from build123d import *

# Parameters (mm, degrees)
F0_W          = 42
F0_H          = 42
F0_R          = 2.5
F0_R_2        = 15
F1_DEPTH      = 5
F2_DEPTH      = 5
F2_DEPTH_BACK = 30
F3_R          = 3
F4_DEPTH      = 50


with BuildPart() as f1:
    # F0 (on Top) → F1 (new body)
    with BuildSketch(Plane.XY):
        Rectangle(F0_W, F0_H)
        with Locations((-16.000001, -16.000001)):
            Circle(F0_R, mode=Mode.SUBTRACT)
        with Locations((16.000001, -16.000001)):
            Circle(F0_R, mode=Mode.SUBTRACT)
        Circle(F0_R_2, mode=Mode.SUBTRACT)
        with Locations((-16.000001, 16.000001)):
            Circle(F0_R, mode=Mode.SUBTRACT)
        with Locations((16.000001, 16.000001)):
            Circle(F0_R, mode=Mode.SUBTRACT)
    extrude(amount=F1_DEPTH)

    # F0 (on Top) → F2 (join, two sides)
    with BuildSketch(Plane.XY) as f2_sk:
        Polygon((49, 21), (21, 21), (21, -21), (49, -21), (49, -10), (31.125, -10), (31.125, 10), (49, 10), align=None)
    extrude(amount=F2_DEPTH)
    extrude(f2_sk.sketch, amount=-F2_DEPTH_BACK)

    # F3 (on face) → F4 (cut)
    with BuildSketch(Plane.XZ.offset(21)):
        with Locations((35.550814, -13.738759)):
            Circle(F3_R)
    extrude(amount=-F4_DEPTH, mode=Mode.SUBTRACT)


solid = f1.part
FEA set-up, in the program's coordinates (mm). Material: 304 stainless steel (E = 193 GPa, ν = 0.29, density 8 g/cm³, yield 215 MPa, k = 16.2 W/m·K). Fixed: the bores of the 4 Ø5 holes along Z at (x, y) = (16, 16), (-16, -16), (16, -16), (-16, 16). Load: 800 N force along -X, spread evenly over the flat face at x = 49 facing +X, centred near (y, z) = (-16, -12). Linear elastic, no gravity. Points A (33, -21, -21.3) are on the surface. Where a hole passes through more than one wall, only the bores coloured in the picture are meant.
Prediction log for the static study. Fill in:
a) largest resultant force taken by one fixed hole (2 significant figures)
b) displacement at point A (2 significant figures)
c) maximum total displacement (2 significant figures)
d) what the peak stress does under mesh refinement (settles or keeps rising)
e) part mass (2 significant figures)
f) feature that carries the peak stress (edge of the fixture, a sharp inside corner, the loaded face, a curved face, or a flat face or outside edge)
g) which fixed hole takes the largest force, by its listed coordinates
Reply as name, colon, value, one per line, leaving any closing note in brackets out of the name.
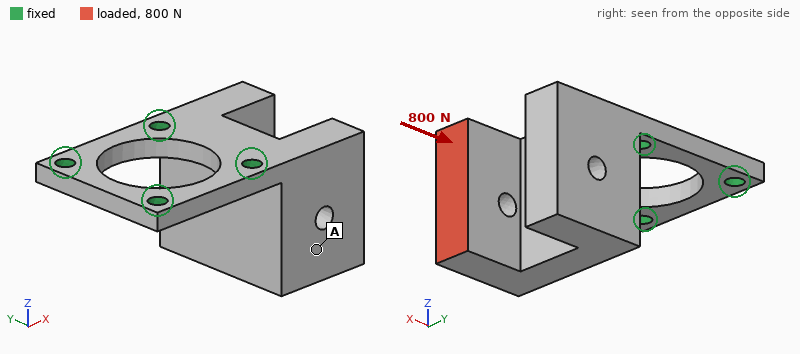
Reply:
largest resultant force taken by one fixed hole: 770 N
displacement at point A: 36 µm
maximum total displacement: 57 µm
what the peak stress does under mesh refinement: keeps rising
part mass: 260 g
feature that carries the peak stress: edge of the fixture
which fixed hole takes the largest force, by its listed coordinates: (16, -16)
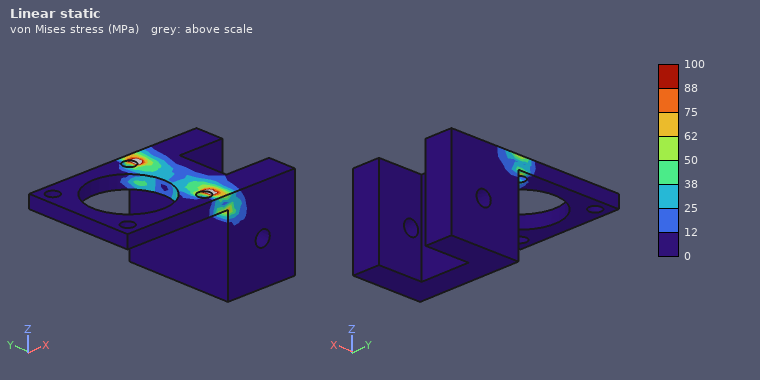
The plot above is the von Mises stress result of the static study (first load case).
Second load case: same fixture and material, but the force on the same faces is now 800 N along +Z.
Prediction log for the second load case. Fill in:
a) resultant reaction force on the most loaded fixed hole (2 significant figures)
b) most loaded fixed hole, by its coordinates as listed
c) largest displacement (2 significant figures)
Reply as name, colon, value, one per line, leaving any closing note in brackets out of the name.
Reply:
resultant reaction force on the most loaded fixed hole: 790 N
most loaded fixed hole, by its coordinates as listed: (16, -16)
largest displacement: 0.11 mm
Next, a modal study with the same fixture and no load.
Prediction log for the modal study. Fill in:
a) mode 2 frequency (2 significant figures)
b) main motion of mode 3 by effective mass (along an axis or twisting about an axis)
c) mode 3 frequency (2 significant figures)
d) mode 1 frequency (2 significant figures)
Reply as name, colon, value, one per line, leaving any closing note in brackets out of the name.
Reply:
mode 2 frequency: 5200 Hz
main motion of mode 3 by effective mass: along Y
mode 3 frequency: 6000 Hz
mode 1 frequency: 1400 Hz
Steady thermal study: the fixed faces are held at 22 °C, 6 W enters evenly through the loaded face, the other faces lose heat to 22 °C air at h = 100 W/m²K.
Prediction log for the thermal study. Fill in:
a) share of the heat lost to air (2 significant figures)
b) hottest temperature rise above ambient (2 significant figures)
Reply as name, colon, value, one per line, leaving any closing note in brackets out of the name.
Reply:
share of the heat lost to air: 80 %
hottest temperature rise above ambient: 24 K
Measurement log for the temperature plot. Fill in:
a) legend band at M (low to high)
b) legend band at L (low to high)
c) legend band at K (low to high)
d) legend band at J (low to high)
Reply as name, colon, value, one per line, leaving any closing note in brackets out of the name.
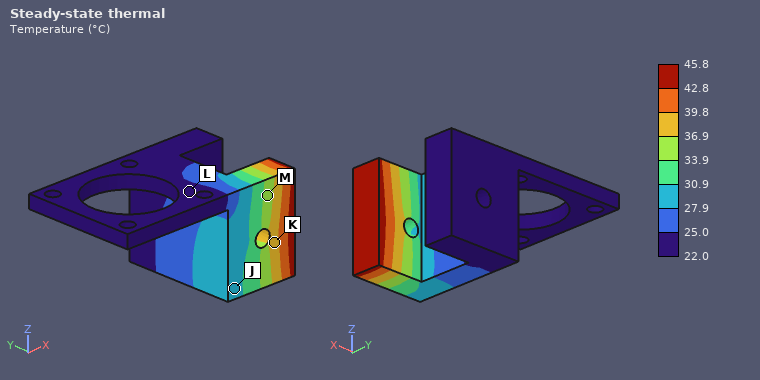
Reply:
legend band at M: 33.9 to 36.9 °C
legend band at L: 22.0 to 25.0 °C
legend band at K: 36.9 to 39.8 °C
legend band at J: 27.9 to 30.9 °C
